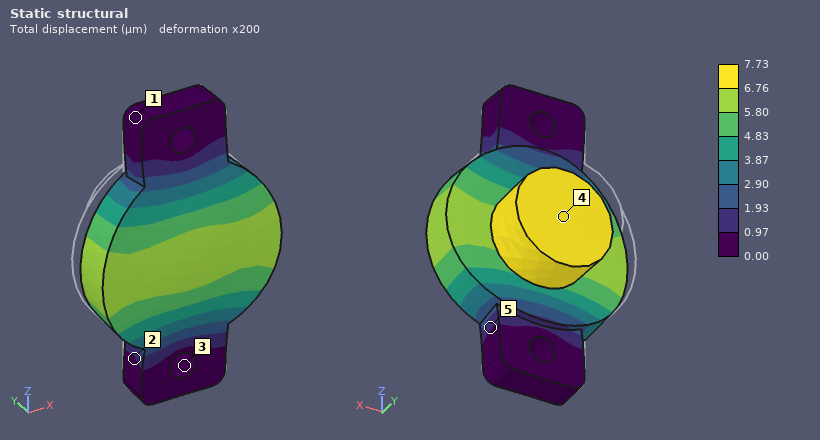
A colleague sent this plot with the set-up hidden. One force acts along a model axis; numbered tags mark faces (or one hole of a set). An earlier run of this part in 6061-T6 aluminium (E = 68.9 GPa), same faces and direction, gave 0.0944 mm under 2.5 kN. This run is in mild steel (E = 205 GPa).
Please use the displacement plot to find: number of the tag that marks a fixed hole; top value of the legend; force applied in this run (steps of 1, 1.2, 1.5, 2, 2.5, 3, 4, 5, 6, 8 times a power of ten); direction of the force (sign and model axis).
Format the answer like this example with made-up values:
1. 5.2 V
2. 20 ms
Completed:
1. 3
2. 7.73 µm
3. 600 N
4. -Y
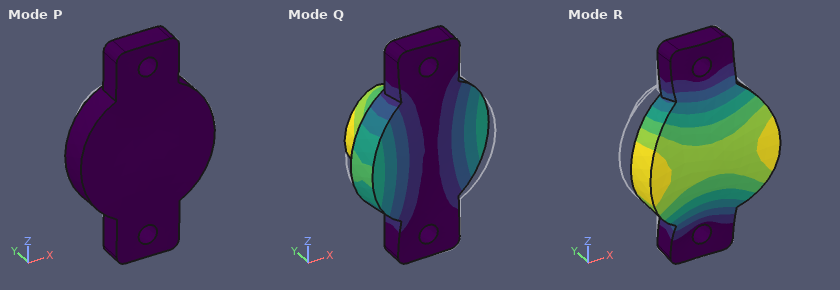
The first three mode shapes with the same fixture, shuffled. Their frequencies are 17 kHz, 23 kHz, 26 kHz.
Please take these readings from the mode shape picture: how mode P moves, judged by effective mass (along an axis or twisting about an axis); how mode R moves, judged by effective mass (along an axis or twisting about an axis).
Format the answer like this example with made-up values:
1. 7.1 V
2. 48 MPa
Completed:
1. along Z
2. along Y
